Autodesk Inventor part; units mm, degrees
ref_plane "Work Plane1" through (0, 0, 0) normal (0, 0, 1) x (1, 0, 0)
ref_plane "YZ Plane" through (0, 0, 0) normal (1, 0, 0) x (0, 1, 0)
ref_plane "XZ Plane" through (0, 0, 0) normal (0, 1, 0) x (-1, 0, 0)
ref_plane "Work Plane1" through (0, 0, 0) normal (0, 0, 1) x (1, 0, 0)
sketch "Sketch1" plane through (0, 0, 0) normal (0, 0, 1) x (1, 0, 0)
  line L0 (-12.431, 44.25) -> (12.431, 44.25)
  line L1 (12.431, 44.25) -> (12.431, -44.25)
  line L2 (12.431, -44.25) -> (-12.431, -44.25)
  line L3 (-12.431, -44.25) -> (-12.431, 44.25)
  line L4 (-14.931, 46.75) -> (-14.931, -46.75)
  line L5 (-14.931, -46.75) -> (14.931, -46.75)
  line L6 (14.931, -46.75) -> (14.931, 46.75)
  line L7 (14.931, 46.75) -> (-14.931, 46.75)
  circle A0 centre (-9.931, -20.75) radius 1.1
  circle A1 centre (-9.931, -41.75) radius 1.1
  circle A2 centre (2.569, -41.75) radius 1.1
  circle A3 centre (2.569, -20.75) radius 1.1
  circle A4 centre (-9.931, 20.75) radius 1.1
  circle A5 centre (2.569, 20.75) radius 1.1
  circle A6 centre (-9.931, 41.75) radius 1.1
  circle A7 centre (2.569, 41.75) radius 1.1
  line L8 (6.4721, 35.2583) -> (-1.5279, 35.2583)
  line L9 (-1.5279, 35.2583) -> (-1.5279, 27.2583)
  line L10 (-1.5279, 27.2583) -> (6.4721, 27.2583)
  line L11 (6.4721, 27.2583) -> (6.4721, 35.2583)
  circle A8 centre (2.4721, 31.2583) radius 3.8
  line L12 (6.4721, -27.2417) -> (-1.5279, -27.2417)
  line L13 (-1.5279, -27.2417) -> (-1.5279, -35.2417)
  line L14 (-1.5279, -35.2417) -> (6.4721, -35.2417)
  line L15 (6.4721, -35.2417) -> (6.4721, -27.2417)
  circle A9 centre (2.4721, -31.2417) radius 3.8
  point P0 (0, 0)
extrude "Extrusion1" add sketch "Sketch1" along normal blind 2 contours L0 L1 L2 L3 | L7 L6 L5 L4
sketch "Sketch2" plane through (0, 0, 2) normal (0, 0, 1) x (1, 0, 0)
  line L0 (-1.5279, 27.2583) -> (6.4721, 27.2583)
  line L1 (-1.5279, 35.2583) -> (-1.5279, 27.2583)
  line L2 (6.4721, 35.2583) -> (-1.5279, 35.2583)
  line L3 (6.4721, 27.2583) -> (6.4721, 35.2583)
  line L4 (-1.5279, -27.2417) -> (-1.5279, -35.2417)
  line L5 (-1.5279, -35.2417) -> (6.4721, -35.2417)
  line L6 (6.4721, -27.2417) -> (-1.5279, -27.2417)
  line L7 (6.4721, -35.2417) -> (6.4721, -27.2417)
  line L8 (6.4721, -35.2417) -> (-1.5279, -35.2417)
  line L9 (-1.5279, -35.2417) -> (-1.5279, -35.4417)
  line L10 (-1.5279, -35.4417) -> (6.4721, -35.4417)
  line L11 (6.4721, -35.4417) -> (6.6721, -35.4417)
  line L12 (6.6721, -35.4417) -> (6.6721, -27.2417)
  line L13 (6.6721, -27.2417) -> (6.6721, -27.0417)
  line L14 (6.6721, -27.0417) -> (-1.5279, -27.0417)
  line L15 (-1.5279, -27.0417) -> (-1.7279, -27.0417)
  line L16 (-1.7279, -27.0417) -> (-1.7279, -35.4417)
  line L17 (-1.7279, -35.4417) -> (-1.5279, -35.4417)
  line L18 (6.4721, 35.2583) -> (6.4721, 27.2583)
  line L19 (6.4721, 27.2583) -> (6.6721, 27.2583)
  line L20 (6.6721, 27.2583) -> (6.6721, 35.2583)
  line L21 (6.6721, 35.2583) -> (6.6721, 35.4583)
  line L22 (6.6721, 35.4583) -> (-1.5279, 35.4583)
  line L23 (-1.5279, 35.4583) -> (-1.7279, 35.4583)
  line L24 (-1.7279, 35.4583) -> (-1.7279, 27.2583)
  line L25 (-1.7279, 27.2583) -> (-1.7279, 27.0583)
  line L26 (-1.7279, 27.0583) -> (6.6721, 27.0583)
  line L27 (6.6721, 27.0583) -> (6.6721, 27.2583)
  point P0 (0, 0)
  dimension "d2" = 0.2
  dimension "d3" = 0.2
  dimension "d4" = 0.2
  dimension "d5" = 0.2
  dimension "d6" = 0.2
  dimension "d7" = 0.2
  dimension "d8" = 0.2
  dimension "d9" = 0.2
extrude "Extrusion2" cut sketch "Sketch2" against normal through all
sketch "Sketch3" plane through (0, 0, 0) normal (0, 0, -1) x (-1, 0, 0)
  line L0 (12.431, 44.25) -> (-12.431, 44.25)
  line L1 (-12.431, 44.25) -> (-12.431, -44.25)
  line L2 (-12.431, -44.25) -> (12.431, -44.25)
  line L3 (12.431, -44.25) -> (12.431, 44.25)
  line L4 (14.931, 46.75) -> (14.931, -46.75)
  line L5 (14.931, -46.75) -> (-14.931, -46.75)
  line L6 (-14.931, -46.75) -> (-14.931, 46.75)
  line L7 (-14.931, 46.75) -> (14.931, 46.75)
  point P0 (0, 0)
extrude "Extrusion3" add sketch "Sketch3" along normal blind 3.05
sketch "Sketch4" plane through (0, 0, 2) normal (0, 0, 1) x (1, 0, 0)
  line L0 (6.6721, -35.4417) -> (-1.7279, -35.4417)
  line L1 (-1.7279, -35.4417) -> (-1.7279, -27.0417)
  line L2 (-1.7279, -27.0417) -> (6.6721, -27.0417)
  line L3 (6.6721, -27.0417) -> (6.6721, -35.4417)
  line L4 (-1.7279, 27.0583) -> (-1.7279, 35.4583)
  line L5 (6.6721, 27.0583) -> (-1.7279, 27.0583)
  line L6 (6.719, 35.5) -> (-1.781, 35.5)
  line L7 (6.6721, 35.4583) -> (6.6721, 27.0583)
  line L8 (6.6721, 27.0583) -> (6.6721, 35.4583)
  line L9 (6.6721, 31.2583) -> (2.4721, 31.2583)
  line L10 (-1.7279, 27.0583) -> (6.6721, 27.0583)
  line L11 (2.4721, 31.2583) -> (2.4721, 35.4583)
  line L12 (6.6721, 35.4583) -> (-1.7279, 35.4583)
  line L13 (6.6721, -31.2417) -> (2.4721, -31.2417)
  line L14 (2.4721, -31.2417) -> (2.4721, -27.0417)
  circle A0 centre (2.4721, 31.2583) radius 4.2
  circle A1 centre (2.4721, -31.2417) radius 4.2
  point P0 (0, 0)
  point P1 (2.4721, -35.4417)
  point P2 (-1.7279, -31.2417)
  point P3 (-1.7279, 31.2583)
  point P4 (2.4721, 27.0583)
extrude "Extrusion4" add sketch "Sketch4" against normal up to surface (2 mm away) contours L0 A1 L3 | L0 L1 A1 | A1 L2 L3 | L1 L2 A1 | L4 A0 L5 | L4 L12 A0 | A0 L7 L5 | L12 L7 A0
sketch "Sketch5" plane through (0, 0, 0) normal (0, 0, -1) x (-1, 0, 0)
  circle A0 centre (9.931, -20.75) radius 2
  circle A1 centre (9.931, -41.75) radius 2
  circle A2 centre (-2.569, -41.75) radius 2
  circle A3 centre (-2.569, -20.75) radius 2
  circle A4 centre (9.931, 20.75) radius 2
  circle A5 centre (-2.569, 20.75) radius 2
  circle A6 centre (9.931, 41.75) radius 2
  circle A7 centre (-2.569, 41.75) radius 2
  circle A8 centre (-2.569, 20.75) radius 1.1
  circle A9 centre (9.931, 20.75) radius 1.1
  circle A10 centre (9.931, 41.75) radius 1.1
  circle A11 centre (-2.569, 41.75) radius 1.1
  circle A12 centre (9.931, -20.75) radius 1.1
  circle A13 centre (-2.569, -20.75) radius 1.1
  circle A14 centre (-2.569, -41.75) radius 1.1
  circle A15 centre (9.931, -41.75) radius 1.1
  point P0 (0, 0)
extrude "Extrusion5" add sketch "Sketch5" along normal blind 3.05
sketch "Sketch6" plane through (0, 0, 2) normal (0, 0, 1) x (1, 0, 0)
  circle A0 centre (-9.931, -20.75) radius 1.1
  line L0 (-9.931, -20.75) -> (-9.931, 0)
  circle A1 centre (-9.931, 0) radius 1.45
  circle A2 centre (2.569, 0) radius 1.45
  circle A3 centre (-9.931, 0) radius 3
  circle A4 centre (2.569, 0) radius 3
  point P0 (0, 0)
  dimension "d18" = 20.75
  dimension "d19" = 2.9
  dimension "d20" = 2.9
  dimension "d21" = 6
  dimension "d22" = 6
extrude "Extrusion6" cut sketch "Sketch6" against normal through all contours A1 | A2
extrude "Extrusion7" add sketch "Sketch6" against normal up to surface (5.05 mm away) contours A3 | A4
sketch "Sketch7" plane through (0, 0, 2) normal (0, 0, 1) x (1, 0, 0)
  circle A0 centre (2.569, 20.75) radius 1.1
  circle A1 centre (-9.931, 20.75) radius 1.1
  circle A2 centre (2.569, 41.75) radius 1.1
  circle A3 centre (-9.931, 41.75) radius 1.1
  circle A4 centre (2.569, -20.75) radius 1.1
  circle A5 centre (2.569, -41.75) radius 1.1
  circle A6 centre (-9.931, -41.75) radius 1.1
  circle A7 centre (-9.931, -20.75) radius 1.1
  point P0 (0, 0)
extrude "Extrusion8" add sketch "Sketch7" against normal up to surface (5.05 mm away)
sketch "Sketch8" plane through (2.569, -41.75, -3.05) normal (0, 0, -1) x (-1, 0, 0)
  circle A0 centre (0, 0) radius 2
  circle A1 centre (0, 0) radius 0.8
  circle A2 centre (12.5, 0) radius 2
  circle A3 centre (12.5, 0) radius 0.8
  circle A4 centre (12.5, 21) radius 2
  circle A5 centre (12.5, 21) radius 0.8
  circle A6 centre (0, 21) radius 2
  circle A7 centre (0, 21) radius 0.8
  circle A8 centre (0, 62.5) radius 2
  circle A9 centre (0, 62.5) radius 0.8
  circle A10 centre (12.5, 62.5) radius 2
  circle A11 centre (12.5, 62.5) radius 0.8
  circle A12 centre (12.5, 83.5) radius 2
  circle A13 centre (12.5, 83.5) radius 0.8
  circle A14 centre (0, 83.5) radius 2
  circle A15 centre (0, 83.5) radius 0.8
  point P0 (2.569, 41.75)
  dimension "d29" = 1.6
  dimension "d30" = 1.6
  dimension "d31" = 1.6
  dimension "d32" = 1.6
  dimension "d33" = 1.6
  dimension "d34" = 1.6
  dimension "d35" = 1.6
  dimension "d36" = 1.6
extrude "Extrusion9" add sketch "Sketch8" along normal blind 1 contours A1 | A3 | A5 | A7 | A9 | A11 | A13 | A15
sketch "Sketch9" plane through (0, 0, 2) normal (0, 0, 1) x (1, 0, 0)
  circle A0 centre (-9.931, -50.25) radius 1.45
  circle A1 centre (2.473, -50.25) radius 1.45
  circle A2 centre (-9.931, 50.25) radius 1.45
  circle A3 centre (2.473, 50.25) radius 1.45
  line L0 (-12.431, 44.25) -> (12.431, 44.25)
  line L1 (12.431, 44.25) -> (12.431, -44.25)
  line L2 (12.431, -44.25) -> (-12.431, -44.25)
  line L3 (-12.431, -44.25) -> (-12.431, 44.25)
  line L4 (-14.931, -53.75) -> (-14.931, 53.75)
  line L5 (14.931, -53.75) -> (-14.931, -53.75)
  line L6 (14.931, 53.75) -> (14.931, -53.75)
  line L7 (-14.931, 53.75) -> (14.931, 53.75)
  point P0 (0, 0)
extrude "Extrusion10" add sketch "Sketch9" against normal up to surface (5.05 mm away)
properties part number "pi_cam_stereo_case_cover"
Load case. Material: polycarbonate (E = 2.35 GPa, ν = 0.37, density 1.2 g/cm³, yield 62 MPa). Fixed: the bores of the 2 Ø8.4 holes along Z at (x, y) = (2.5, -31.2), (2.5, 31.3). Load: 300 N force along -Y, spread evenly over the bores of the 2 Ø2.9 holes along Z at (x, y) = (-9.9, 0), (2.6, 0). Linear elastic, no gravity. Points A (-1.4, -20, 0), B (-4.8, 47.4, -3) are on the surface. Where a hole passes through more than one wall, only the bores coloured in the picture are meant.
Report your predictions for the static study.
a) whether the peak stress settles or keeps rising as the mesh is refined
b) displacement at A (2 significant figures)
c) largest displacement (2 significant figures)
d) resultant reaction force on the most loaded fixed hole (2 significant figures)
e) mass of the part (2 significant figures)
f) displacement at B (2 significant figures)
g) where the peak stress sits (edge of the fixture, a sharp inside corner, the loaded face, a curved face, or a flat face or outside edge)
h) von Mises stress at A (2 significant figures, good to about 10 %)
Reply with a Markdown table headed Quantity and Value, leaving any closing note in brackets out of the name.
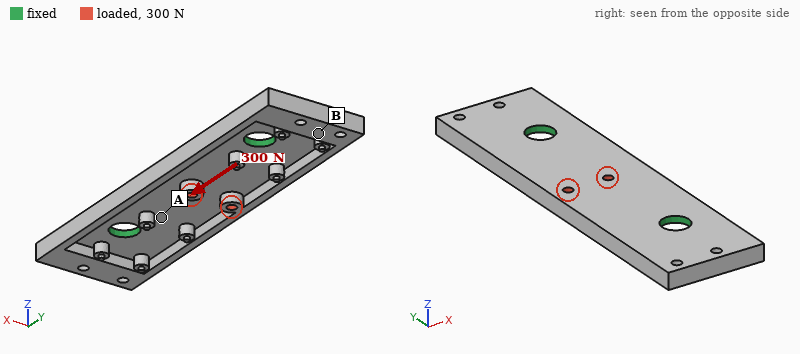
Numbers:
| Quantity | Value |
|---|---|
| whether the peak stress settles or keeps rising as the mesh is refined | keeps rising |
| displacement at A | 0.029 mm |
| largest displacement | 0.13 mm |
| resultant reaction force on the most loaded fixed hole | 150 N |
| mass of the part | 11 g |
| displacement at B | 0.027 mm |
| where the peak stress sits | a sharp inside corner |
| von Mises stress at A | 3.6 MPa |
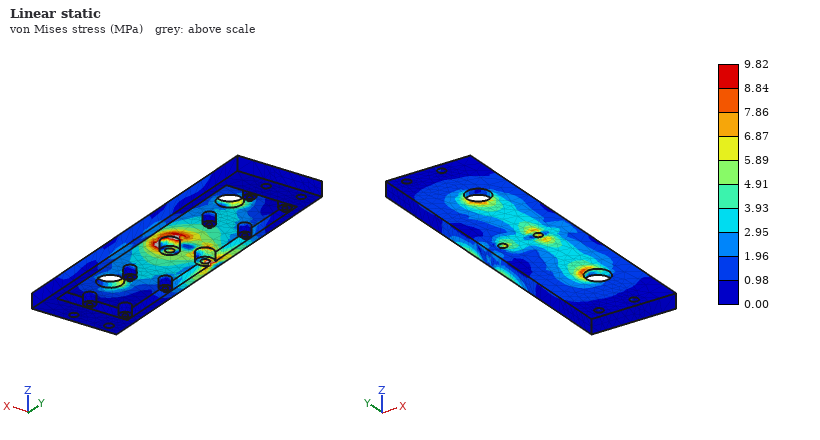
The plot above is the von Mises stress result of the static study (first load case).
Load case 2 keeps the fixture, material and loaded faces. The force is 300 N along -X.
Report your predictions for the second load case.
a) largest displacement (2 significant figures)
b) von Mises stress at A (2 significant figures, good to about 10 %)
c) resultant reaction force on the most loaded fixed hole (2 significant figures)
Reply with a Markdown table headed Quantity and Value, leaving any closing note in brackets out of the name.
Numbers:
| Quantity | Value |
|---|---|
| largest displacement | 0.80 mm |
| von Mises stress at A | 12 MPa |
| resultant reaction force on the most loaded fixed hole | 150 N |
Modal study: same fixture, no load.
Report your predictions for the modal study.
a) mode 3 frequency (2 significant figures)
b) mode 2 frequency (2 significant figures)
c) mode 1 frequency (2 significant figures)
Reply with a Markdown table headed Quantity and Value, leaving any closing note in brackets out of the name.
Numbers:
| Quantity | Value |
|---|---|
| mode 3 frequency | 1100 Hz |
| mode 2 frequency | 1100 Hz |
| mode 1 frequency | 910 Hz |
